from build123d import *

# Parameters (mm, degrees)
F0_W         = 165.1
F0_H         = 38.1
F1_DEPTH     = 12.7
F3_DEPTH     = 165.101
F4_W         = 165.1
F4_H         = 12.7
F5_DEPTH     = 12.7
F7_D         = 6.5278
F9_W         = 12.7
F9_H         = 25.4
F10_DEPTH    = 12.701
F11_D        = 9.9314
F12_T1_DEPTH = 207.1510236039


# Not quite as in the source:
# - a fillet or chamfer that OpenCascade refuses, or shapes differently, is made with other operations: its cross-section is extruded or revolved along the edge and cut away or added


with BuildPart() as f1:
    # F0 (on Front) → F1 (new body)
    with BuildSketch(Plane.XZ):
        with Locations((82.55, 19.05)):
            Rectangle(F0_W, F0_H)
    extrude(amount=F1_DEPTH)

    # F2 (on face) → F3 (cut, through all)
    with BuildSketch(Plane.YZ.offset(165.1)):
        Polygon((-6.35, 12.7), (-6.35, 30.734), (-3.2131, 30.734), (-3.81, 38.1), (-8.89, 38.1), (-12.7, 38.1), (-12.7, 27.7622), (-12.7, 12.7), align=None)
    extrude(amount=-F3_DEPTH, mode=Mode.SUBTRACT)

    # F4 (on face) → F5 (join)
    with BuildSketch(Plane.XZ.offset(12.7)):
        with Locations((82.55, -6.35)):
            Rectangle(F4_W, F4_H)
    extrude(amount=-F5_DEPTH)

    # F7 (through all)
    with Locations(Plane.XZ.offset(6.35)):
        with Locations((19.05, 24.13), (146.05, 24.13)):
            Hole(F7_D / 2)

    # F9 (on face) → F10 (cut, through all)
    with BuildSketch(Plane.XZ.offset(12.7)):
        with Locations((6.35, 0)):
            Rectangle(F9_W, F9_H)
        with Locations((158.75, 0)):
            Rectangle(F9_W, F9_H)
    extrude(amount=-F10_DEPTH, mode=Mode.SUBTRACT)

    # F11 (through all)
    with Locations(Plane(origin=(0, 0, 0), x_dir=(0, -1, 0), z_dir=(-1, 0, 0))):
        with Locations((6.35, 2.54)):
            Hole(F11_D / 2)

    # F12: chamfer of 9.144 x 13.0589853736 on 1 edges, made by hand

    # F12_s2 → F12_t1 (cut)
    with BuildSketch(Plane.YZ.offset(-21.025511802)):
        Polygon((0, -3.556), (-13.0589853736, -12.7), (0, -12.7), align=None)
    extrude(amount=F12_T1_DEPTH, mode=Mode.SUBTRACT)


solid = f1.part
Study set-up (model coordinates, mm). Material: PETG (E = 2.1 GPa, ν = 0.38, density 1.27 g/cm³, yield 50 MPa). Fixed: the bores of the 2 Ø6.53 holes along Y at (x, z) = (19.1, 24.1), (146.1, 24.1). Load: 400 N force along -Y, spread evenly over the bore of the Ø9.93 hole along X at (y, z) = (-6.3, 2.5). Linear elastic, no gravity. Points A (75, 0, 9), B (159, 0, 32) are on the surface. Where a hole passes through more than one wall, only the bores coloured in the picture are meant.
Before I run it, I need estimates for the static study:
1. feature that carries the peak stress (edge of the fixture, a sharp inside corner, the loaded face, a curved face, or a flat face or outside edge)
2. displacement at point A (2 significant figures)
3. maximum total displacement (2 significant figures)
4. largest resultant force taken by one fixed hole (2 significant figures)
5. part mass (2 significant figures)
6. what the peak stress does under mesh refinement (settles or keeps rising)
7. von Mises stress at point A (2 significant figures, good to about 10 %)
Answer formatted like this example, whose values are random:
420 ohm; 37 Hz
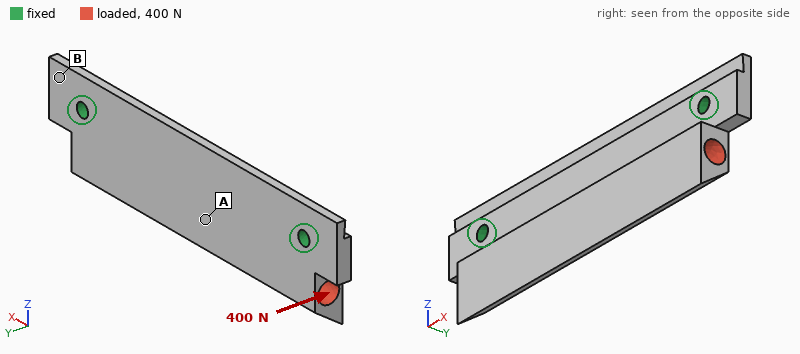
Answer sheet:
edge of the fixture; 1.0 mm; 1.9 mm; 210 N; 62 g; keeps rising; 5.1 MPa
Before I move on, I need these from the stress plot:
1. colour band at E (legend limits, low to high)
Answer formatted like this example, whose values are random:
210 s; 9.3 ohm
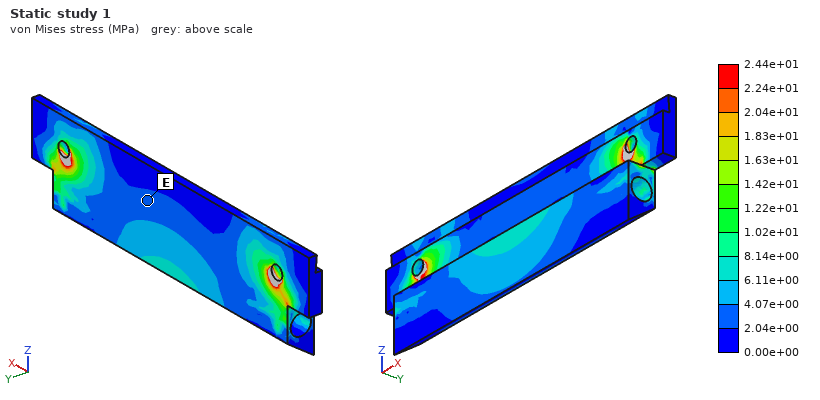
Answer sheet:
2.04e+00 to 4.07e+00 MPa
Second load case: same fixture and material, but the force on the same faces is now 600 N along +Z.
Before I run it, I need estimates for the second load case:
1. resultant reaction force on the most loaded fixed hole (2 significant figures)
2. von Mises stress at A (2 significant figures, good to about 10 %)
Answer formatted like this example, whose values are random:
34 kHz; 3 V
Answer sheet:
340 N; 2.1 MPa
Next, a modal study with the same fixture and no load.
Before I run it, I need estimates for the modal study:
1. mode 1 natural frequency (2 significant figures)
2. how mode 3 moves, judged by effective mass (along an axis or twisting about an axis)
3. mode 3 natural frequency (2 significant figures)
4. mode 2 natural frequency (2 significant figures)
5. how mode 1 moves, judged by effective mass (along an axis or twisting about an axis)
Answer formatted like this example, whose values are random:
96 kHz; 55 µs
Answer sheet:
480 Hz; twisting about Z; 1200 Hz; 770 Hz; along Y
